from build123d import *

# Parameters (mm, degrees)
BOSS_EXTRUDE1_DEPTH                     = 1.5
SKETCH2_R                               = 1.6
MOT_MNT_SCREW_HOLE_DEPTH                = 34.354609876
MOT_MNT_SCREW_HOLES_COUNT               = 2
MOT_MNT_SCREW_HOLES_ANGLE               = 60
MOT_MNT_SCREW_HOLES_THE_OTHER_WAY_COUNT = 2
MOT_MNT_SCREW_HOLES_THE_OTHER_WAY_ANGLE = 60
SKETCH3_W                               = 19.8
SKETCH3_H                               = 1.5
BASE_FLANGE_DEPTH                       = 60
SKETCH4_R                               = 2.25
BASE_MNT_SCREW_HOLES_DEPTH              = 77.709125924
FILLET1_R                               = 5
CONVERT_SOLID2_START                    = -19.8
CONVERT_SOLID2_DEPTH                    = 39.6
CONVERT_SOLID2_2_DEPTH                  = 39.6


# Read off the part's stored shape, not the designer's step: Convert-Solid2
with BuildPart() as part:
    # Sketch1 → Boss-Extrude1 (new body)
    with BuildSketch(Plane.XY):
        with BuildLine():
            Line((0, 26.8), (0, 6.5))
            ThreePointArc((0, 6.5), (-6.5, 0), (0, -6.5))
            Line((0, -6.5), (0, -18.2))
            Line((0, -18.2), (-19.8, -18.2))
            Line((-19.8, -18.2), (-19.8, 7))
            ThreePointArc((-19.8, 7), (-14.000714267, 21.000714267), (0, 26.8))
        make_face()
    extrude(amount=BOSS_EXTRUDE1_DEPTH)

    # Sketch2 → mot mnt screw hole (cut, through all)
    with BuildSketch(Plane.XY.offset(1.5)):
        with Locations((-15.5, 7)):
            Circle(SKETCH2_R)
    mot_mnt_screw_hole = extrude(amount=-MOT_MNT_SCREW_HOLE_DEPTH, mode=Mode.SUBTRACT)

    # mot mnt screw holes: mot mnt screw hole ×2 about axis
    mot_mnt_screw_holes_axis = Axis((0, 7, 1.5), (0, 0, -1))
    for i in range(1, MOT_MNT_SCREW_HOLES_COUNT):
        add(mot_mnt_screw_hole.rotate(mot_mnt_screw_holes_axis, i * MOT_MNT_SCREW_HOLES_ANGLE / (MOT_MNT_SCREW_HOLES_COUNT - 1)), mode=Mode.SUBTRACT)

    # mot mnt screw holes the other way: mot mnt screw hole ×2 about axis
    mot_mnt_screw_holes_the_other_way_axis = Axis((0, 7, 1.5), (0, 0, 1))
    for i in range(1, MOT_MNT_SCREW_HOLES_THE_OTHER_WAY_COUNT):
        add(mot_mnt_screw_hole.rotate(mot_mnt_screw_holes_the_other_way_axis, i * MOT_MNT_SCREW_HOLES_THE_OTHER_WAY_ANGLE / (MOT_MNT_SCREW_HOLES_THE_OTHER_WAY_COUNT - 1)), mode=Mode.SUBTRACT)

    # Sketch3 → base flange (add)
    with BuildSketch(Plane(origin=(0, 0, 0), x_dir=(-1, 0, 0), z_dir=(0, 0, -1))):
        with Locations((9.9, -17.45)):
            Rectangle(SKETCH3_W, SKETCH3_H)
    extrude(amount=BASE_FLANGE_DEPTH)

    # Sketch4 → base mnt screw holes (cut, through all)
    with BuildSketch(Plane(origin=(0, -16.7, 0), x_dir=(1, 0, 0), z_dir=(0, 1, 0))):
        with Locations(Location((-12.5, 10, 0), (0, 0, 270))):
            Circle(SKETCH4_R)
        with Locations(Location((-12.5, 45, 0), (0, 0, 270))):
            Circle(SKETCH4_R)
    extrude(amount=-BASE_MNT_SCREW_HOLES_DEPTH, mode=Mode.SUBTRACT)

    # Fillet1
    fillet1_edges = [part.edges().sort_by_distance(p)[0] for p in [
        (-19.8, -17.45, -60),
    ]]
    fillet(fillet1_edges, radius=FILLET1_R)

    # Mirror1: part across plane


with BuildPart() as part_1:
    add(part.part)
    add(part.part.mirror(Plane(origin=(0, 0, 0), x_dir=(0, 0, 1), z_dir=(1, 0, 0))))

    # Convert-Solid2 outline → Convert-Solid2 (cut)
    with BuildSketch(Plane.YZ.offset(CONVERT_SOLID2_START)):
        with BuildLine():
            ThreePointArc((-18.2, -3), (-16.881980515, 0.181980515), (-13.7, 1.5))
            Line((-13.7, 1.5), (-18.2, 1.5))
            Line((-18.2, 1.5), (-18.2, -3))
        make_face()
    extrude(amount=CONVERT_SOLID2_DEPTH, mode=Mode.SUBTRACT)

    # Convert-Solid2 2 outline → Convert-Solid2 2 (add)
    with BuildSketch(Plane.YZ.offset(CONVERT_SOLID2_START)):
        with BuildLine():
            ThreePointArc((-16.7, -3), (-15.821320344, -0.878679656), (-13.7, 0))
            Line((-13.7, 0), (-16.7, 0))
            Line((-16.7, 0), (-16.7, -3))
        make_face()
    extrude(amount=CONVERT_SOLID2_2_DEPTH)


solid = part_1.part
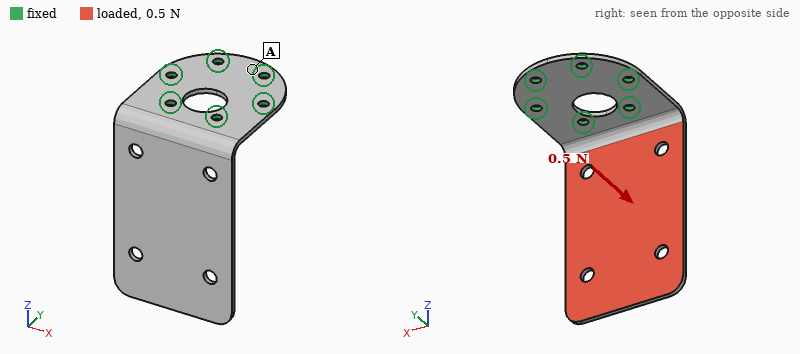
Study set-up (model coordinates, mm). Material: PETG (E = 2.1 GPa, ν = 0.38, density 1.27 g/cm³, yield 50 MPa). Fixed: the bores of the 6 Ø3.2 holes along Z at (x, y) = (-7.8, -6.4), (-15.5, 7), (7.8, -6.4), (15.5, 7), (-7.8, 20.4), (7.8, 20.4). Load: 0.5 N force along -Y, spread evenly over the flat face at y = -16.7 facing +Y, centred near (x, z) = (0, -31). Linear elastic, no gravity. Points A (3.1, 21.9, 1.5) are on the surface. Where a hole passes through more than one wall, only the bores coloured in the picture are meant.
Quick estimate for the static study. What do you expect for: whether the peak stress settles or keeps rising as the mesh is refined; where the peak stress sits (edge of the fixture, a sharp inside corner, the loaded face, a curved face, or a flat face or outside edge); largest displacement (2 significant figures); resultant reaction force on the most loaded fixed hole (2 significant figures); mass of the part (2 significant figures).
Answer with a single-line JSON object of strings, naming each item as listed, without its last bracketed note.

{"whether the peak stress settles or keeps rising as the mesh is refined": "keeps rising", "where the peak stress sits": "edge of the fixture", "largest displacement": "0.98 mm", "resultant reaction force on the most loaded fixed hole": "0.31 N", "mass of the part": "7.0 g"}
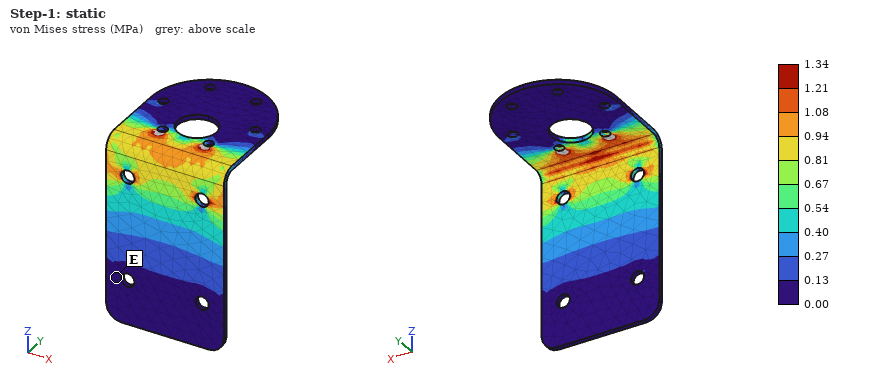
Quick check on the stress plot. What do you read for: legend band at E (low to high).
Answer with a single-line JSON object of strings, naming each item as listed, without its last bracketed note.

{"legend band at E": "0.00 to 0.13 MPa"}
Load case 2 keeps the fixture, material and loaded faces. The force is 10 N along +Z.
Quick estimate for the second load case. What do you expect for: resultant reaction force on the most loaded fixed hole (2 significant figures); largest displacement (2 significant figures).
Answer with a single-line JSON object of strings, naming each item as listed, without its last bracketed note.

{"resultant reaction force on the most loaded fixed hole": "5.8 N", "largest displacement": "0.92 mm"}
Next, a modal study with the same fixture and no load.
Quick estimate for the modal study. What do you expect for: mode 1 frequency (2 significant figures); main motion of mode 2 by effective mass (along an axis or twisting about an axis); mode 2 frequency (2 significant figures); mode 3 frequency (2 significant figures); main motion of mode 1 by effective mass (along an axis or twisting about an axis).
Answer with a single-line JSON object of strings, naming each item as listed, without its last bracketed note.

{"mode 1 frequency": "69 Hz", "main motion of mode 2 by effective mass": "along X", "mode 2 frequency": "200 Hz", "mode 3 frequency": "300 Hz", "main motion of mode 1 by effective mass": "along Y"}
